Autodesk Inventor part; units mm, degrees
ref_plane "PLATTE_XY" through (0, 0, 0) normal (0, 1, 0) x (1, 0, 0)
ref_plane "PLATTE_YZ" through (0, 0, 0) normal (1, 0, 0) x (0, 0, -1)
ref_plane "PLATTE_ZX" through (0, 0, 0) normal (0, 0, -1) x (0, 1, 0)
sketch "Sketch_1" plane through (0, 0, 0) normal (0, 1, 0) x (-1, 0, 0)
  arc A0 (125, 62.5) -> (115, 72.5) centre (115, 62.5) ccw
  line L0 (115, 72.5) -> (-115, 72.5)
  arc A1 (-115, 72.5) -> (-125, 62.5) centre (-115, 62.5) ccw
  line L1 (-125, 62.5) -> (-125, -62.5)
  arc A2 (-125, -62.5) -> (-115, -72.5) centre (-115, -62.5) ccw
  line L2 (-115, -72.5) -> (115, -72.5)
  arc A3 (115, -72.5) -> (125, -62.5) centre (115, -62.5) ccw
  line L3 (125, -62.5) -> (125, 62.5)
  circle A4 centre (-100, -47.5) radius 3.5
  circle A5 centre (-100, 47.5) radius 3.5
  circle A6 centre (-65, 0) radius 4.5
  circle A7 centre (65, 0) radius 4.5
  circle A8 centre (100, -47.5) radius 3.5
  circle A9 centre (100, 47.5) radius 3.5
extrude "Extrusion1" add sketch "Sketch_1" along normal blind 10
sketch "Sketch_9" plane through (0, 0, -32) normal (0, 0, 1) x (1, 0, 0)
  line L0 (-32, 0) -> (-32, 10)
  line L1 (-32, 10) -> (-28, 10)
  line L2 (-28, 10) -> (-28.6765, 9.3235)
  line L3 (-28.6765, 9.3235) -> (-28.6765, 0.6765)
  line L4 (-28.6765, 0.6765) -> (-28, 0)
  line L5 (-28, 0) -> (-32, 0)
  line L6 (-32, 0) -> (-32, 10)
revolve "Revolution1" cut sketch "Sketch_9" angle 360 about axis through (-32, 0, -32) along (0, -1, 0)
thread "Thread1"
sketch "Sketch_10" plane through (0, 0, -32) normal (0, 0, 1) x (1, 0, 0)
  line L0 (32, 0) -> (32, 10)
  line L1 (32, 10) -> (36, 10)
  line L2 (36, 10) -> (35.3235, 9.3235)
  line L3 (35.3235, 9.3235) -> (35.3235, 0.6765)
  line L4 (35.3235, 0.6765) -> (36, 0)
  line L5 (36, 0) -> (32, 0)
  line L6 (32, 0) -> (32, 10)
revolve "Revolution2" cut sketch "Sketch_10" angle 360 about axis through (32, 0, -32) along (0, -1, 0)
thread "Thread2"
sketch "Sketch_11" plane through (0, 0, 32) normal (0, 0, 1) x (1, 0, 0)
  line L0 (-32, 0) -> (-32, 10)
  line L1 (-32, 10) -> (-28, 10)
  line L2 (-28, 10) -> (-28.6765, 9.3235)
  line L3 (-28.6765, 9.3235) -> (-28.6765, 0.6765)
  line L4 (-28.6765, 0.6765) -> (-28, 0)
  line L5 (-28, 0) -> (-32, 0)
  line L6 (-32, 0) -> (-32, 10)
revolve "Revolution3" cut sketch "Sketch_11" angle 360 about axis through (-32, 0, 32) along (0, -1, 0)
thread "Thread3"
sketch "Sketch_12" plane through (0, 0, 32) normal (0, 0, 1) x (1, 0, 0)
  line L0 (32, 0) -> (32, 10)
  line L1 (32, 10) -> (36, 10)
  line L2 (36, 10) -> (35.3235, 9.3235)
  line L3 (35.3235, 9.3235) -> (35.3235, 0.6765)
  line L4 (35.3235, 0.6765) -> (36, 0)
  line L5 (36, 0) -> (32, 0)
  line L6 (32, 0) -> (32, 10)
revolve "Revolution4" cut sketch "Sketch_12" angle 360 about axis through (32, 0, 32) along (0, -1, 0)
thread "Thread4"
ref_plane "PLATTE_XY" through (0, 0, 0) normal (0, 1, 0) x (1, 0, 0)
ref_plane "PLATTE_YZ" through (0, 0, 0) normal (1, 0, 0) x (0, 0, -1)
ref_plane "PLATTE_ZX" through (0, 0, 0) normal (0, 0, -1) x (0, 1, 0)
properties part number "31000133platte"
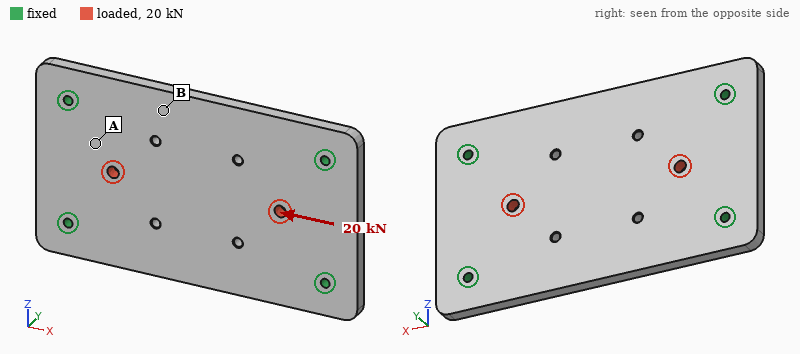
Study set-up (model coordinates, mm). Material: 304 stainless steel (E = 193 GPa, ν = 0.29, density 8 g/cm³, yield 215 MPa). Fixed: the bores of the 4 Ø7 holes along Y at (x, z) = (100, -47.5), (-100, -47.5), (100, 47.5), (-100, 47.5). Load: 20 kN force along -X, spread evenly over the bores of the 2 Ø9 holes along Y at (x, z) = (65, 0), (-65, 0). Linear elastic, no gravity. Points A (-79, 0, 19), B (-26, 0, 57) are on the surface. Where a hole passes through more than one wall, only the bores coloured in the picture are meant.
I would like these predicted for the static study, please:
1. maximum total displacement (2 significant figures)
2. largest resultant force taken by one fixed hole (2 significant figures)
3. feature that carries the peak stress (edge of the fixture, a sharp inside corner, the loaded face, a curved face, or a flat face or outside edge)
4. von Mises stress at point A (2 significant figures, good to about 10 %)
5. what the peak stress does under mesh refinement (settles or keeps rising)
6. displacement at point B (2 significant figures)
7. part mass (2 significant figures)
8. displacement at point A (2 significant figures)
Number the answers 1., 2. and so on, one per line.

1. 6.3 µm
2. 5.1 kN
3. a sharp inside corner
4. 12 MPa
5. keeps rising
6. 2.4 µm
7. 2.9 kg
8. 3.5 µm
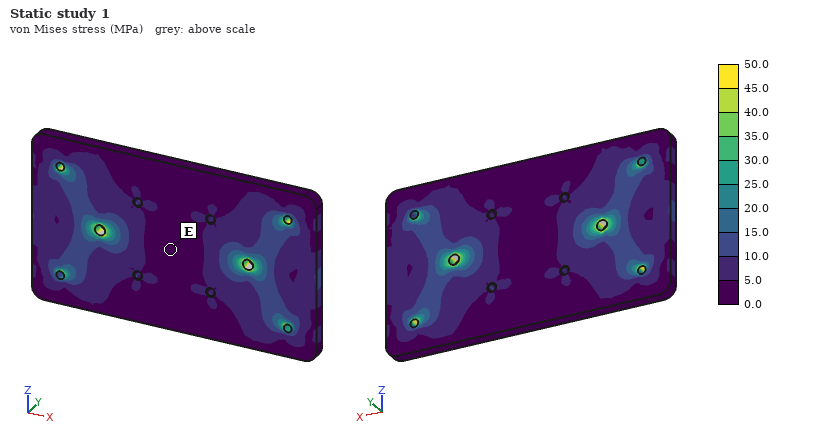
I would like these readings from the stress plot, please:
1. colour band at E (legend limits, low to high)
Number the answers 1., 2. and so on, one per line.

1. 0.0 to 5.0 MPa
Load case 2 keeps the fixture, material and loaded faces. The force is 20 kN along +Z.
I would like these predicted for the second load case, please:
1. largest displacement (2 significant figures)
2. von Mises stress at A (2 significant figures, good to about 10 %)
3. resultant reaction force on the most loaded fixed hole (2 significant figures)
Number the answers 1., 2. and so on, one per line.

1. 7.6 µm
2. 18 MPa
3. 5.6 kN
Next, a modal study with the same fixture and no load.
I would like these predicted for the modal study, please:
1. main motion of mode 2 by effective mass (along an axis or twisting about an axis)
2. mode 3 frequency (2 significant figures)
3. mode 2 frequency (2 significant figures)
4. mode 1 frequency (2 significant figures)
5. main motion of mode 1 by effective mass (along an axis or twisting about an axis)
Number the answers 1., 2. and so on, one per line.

1. twisting about X
2. 2900 Hz
3. 1600 Hz
4. 1100 Hz
5. along Y
